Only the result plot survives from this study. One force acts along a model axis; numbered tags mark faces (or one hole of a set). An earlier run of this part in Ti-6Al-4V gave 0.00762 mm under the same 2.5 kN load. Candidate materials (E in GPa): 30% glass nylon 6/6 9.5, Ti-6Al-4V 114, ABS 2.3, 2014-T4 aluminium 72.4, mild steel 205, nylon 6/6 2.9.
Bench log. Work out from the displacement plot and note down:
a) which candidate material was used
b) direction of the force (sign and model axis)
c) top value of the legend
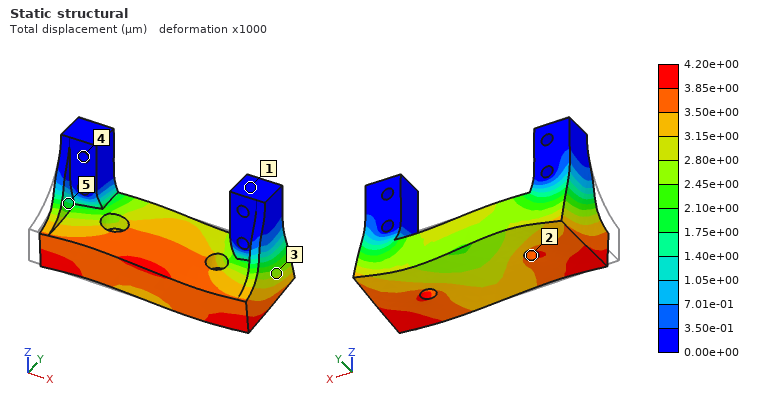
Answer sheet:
mild steel
+X
4.20e+00 µm
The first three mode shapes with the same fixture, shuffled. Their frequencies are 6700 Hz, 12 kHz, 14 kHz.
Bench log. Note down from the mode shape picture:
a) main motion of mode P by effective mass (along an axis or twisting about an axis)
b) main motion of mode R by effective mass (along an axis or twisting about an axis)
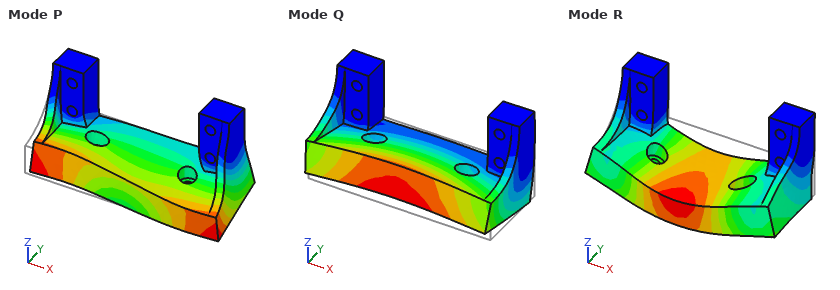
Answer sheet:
along X
along Y
